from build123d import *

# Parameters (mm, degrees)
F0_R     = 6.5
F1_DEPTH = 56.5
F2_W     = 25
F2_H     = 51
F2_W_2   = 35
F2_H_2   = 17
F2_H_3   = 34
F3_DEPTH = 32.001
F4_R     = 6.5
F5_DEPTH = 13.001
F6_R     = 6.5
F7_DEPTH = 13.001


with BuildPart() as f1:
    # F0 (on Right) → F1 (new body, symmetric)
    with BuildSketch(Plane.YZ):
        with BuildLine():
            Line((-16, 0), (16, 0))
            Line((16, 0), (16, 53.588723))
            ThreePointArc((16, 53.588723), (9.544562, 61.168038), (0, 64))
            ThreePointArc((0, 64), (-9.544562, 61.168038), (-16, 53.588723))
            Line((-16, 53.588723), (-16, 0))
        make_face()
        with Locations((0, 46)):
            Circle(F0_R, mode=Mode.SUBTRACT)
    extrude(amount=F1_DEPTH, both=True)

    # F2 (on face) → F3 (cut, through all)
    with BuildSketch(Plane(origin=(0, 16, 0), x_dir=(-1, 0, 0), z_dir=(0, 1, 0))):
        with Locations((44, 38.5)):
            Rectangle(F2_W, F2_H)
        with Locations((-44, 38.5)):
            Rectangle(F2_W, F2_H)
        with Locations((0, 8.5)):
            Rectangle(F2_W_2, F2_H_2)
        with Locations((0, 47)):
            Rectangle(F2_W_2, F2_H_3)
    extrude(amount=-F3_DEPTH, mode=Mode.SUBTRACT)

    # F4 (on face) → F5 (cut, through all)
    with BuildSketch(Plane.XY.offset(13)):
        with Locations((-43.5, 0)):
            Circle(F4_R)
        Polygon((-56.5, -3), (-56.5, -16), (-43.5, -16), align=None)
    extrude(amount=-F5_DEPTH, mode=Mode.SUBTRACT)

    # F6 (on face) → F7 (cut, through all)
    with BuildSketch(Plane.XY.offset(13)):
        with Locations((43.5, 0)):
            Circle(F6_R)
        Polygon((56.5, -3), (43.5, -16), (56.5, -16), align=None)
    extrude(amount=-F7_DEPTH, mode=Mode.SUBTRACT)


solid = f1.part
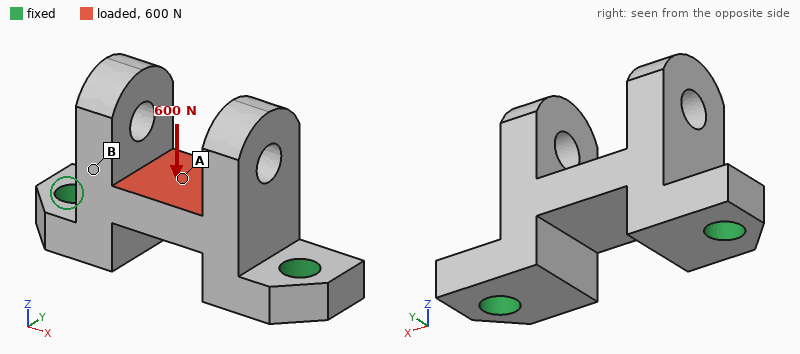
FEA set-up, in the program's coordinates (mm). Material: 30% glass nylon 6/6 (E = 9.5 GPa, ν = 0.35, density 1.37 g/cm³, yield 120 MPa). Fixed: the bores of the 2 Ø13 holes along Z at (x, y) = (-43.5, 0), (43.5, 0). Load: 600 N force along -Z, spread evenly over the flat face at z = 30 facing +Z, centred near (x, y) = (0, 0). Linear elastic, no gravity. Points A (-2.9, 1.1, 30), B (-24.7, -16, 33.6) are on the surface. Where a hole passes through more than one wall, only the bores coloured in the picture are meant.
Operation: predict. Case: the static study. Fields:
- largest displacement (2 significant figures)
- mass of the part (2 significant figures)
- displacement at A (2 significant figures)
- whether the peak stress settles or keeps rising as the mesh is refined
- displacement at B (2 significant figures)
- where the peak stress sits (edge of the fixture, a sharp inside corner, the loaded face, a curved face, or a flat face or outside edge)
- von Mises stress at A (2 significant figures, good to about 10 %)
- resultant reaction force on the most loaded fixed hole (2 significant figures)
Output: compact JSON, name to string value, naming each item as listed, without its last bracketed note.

{"largest displacement": "16 µm", "mass of the part": "110 g", "displacement at A": "13 µm", "whether the peak stress settles or keeps rising as the mesh is refined": "keeps rising", "displacement at B": "7.0 µm", "where the peak stress sits": "edge of the fixture", "von Mises stress at A": "2.4 MPa", "resultant reaction force on the most loaded fixed hole": "430 N"}
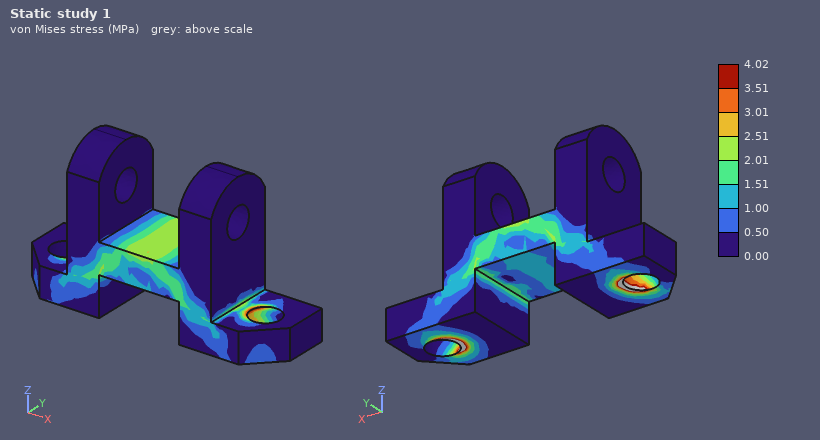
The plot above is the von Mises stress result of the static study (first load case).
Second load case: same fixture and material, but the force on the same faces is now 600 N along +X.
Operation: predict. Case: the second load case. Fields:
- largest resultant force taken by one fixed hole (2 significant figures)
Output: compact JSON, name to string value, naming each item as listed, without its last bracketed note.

{"largest resultant force taken by one fixed hole": "350 N"}
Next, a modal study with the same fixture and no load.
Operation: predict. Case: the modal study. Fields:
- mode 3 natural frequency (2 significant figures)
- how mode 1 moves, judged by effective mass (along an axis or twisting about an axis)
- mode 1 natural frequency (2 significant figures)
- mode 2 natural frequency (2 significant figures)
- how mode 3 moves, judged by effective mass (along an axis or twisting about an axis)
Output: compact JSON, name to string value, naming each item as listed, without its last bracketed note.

{"mode 3 natural frequency": "2900 Hz", "how mode 1 moves, judged by effective mass": "along Y", "mode 1 natural frequency": "1800 Hz", "mode 2 natural frequency": "2700 Hz", "how mode 3 moves, judged by effective mass": "along X"}
